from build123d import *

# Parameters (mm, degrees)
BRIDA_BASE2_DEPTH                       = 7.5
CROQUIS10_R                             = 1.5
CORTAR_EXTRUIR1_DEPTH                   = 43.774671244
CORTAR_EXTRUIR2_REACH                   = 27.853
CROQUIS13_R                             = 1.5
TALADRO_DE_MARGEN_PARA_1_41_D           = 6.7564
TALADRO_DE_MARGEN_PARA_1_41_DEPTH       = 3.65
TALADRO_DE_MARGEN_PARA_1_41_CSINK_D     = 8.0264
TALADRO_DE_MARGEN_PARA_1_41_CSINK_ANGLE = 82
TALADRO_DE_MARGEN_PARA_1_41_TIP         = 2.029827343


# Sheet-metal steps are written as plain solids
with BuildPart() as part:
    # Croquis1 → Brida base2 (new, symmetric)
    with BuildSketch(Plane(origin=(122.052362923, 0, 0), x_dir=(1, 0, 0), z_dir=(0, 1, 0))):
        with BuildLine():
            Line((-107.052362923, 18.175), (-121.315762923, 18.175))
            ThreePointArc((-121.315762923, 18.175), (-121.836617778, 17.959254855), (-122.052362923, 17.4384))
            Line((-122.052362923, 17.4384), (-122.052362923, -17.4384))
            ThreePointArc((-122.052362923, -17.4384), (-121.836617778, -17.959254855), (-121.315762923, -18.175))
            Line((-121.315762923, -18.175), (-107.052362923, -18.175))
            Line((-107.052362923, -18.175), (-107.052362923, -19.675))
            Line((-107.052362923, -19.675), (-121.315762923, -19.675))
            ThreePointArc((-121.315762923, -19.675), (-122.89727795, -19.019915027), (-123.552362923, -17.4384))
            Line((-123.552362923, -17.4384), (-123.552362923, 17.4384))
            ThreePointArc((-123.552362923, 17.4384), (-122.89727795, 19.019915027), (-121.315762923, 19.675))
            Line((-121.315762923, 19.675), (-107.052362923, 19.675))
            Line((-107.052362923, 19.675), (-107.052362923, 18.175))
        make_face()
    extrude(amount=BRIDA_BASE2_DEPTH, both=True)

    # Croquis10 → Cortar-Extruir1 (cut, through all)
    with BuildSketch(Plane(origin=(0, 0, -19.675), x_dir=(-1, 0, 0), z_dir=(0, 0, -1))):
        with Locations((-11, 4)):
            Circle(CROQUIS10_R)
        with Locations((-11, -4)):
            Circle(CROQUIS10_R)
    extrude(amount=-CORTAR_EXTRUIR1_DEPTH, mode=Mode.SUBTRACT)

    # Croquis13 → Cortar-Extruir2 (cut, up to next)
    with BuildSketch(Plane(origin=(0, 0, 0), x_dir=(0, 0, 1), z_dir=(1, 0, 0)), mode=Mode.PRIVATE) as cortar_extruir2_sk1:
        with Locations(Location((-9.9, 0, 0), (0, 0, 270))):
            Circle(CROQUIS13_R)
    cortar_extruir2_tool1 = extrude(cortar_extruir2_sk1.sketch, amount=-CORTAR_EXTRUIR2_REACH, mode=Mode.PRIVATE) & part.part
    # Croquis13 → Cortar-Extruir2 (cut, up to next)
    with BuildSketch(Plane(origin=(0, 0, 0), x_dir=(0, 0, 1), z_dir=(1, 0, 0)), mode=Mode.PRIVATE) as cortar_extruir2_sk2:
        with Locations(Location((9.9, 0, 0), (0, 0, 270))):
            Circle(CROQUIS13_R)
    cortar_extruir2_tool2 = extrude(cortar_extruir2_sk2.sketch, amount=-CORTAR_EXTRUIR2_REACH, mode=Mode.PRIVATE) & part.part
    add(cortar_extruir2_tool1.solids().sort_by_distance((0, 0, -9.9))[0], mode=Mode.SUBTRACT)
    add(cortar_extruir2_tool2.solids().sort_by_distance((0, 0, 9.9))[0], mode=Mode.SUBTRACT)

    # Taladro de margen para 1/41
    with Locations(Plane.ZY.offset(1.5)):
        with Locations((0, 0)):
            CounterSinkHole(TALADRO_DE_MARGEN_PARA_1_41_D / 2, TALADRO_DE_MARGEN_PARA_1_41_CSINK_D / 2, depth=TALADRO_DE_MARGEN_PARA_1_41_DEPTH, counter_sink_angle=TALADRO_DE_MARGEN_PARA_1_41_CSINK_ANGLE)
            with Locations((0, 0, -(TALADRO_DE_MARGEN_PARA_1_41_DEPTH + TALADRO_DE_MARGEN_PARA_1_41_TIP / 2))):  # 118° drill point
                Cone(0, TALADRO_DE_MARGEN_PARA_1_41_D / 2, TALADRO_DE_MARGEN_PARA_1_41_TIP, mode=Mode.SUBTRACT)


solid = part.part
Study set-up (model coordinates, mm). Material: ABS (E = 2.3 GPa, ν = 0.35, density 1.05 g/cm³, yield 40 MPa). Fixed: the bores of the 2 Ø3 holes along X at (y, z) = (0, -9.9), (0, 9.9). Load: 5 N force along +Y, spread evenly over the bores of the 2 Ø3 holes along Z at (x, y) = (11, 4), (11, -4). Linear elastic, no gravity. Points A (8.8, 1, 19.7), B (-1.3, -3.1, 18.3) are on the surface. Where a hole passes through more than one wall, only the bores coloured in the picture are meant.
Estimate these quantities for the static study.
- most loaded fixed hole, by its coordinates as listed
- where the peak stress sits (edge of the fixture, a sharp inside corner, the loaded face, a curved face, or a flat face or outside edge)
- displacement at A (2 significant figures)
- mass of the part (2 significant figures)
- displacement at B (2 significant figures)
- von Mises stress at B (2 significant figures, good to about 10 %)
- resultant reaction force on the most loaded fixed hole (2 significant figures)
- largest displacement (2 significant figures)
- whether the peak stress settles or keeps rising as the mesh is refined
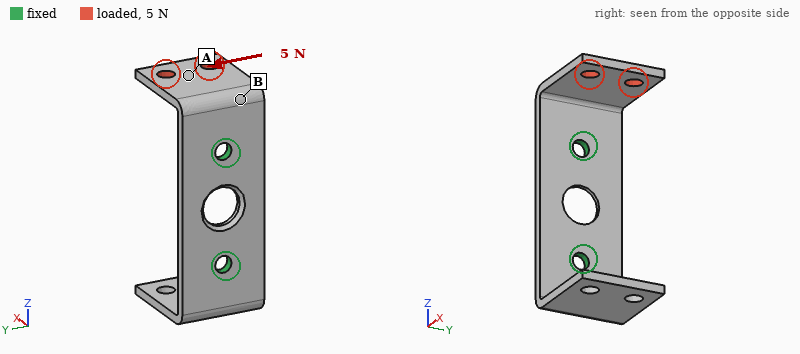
(0, 9.9)
edge of the fixture
0.26 mm
1.5 g
0.082 mm
4.3 MPa
6.3 N
0.50 mm
keeps rising
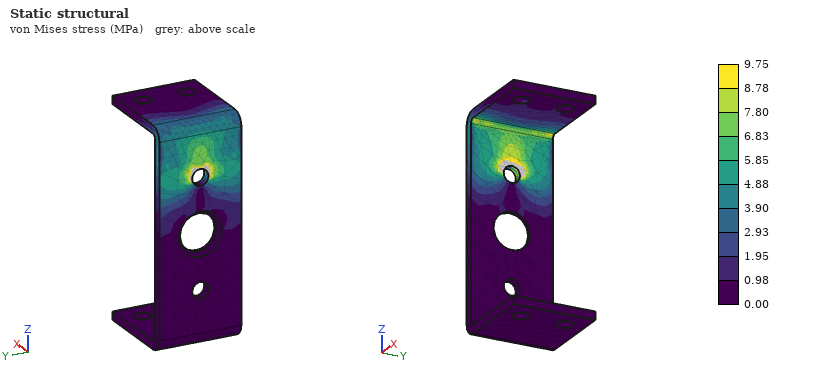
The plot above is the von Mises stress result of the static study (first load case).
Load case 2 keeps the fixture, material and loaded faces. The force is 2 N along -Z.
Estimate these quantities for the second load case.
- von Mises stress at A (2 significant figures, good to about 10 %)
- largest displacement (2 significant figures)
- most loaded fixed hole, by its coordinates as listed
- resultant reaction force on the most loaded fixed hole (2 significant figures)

0.80 MPa
0.46 mm
(0, 9.9)
1.8 N
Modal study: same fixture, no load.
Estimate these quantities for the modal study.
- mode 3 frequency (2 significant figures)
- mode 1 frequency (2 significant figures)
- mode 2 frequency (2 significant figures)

1200 Hz
830 Hz
830 Hz
